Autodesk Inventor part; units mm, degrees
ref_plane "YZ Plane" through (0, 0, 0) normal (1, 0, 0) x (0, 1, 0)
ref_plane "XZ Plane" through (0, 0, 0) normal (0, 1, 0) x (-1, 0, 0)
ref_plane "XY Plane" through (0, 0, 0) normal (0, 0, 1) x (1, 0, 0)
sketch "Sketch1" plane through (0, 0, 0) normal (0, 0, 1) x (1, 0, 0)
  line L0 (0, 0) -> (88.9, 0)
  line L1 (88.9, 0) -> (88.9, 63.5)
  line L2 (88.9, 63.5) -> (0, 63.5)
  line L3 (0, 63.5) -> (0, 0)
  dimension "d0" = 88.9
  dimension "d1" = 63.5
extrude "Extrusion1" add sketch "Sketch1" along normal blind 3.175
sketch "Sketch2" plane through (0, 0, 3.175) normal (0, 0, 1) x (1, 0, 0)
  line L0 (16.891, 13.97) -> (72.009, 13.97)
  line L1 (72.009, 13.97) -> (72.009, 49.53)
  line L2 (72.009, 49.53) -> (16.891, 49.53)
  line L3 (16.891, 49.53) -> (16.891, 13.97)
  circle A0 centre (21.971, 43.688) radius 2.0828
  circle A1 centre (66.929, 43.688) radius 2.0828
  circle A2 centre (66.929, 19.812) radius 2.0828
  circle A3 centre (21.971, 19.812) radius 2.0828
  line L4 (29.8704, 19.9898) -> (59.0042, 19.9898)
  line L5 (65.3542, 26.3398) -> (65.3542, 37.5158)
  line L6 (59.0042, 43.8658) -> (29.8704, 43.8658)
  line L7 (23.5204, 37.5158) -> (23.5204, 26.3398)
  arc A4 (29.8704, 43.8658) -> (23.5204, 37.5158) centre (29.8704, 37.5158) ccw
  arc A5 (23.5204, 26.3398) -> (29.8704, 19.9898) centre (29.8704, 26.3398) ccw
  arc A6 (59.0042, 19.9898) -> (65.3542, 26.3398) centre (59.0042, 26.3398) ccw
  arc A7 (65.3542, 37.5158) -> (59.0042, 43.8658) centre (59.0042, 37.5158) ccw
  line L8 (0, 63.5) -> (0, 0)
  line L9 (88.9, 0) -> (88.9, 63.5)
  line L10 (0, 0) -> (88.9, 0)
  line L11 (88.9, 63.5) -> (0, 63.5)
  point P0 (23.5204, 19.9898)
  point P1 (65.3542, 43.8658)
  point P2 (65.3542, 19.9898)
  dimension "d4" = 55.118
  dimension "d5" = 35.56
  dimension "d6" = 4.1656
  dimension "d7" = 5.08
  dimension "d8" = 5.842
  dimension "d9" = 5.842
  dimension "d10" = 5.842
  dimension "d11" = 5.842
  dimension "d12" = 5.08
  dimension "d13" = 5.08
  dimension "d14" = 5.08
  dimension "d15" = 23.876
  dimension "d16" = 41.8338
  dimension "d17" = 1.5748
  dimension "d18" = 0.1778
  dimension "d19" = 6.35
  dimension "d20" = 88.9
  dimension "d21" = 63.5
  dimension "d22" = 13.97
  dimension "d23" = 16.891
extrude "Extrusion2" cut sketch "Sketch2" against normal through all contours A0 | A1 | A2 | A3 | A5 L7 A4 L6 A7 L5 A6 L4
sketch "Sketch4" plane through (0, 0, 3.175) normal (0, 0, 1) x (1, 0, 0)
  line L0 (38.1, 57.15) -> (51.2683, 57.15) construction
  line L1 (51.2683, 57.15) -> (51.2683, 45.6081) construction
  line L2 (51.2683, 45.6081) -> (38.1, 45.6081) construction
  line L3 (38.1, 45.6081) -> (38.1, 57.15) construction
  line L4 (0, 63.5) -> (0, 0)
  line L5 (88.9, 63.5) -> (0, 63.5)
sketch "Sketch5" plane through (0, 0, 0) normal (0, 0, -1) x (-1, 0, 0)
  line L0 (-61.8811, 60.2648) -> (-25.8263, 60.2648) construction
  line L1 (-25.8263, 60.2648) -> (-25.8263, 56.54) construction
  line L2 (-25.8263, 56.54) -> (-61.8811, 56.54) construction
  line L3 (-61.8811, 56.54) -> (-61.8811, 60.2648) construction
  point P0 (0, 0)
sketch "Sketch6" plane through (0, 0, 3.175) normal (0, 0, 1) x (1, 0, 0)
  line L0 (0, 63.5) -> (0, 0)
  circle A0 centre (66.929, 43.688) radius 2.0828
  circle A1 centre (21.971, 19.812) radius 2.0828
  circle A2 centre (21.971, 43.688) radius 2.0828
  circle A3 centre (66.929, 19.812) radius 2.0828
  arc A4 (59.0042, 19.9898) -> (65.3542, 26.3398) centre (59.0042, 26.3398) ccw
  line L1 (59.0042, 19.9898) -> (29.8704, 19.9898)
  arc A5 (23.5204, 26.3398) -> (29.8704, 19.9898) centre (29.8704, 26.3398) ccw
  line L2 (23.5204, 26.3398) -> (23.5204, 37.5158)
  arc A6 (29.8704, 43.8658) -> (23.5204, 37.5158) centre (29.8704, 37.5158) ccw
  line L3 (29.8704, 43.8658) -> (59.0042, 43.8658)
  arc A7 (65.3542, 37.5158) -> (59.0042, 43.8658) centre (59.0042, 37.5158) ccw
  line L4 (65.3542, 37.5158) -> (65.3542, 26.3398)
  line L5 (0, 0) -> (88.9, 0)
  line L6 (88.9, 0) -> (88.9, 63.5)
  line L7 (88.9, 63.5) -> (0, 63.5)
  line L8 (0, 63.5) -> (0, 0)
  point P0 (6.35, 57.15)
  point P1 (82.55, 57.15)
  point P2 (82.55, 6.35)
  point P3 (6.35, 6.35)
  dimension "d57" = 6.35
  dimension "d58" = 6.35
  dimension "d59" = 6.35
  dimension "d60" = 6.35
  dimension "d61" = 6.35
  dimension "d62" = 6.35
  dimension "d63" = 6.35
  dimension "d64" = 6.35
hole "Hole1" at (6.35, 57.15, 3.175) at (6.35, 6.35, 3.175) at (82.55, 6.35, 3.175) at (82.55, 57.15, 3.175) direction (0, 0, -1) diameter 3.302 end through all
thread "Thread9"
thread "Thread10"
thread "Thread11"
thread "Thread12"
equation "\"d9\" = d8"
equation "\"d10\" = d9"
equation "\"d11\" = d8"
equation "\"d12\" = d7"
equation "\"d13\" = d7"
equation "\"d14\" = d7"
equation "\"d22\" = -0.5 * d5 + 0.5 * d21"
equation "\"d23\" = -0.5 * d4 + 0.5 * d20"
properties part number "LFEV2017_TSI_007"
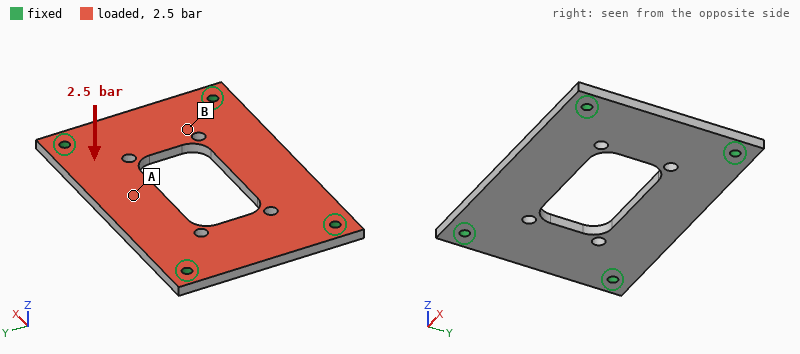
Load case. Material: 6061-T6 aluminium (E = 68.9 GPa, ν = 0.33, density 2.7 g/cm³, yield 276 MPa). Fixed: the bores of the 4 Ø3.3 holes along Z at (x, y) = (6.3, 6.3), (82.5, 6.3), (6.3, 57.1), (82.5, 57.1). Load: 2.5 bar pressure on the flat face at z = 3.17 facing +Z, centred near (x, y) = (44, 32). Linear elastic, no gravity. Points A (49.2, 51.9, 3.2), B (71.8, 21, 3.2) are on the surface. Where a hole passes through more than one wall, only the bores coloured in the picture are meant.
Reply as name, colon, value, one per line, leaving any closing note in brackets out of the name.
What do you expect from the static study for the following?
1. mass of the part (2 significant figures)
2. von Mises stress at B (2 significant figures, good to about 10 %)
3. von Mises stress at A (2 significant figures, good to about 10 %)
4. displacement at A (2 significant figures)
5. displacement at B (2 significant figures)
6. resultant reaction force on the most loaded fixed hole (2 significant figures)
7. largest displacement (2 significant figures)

mass of the part: 39 g
von Mises stress at B: 17 MPa
von Mises stress at A: 35 MPa
displacement at A: 0.14 mm
displacement at B: 0.068 mm
resultant reaction force on the most loaded fixed hole: 290 N
largest displacement: 0.17 mm
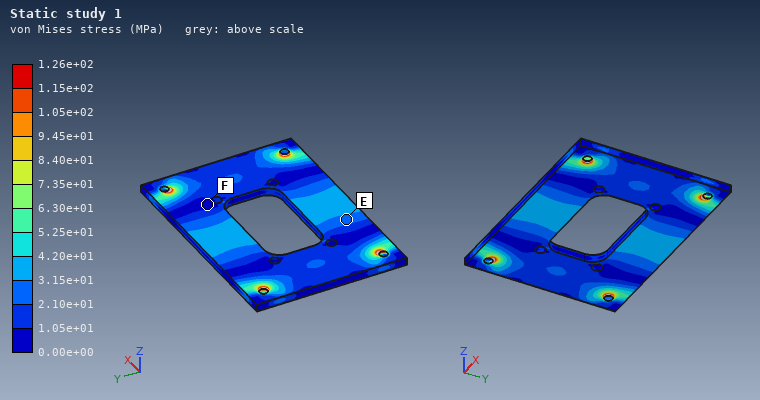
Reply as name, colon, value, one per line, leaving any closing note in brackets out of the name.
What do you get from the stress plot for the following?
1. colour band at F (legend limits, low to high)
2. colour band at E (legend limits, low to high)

colour band at F: 0.00e+00 to 1.05e+01 MPa
colour band at E: 2.10e+01 to 3.15e+01 MPa
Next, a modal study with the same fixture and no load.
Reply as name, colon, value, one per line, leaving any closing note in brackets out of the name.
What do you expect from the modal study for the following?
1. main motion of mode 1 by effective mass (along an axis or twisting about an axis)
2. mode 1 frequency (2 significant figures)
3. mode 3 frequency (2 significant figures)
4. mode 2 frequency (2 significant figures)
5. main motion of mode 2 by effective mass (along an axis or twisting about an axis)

main motion of mode 1 by effective mass: along Z
mode 1 frequency: 2600 Hz
mode 3 frequency: 5200 Hz
mode 2 frequency: 3200 Hz
main motion of mode 2 by effective mass: twisting about X
